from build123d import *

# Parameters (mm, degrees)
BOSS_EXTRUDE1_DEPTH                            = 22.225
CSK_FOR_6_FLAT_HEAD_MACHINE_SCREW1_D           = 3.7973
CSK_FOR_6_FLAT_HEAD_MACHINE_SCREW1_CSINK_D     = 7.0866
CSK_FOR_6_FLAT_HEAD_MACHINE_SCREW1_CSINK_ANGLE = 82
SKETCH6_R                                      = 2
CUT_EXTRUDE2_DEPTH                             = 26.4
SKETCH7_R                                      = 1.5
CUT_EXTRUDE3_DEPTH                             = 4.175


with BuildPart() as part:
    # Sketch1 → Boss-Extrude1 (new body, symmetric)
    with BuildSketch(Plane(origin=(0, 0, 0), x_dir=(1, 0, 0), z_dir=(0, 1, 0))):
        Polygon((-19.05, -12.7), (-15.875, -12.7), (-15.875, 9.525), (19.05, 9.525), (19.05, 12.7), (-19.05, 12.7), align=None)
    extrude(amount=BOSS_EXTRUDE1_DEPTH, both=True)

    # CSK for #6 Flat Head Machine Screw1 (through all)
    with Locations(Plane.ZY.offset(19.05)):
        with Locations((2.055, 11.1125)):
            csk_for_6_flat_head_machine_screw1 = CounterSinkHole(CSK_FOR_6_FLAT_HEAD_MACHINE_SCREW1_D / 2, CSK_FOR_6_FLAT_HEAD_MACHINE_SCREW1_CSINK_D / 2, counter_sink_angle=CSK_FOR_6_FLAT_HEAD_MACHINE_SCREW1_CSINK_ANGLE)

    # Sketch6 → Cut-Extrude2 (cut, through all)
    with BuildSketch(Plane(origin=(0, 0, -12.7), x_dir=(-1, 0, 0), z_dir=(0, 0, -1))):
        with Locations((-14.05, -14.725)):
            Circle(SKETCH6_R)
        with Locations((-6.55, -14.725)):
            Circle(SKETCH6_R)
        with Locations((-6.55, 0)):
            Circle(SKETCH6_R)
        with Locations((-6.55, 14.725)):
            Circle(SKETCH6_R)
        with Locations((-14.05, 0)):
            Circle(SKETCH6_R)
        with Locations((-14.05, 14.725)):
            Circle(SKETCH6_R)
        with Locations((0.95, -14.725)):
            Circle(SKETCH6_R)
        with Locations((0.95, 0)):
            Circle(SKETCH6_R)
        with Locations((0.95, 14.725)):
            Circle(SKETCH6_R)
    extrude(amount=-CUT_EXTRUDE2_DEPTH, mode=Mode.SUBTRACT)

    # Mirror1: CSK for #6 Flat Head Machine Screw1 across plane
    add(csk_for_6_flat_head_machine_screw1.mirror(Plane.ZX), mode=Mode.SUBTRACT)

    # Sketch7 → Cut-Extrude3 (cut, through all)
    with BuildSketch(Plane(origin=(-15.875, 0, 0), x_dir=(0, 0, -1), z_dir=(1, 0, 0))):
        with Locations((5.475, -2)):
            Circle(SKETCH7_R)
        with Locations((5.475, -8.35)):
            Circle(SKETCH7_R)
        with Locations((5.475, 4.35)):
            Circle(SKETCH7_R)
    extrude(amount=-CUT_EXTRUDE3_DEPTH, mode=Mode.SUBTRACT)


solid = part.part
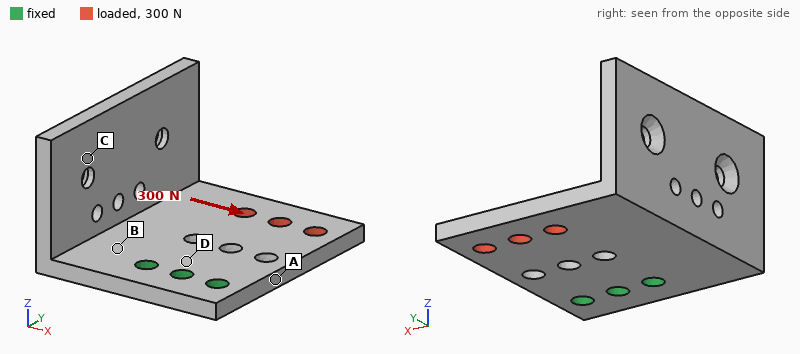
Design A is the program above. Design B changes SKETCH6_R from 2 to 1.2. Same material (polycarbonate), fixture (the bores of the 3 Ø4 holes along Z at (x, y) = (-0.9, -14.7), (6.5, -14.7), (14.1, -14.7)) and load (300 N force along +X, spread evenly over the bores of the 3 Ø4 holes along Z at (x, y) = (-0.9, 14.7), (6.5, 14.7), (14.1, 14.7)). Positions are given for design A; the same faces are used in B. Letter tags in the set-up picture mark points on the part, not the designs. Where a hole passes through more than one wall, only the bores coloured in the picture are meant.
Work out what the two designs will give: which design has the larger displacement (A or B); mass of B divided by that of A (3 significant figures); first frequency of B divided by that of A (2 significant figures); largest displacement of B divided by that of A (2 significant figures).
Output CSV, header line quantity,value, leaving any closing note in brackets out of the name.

quantity,value
which design has the larger displacement,B
mass of B divided by that of A,1.03
first frequency of B divided by that of A,0.93
largest displacement of B divided by that of A,1.1
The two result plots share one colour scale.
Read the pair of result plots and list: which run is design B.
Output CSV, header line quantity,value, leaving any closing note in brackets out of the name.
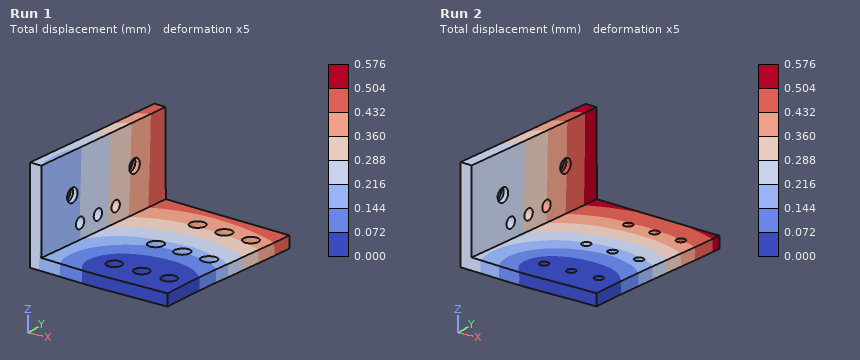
quantity,value
which run is design B,Run 2
